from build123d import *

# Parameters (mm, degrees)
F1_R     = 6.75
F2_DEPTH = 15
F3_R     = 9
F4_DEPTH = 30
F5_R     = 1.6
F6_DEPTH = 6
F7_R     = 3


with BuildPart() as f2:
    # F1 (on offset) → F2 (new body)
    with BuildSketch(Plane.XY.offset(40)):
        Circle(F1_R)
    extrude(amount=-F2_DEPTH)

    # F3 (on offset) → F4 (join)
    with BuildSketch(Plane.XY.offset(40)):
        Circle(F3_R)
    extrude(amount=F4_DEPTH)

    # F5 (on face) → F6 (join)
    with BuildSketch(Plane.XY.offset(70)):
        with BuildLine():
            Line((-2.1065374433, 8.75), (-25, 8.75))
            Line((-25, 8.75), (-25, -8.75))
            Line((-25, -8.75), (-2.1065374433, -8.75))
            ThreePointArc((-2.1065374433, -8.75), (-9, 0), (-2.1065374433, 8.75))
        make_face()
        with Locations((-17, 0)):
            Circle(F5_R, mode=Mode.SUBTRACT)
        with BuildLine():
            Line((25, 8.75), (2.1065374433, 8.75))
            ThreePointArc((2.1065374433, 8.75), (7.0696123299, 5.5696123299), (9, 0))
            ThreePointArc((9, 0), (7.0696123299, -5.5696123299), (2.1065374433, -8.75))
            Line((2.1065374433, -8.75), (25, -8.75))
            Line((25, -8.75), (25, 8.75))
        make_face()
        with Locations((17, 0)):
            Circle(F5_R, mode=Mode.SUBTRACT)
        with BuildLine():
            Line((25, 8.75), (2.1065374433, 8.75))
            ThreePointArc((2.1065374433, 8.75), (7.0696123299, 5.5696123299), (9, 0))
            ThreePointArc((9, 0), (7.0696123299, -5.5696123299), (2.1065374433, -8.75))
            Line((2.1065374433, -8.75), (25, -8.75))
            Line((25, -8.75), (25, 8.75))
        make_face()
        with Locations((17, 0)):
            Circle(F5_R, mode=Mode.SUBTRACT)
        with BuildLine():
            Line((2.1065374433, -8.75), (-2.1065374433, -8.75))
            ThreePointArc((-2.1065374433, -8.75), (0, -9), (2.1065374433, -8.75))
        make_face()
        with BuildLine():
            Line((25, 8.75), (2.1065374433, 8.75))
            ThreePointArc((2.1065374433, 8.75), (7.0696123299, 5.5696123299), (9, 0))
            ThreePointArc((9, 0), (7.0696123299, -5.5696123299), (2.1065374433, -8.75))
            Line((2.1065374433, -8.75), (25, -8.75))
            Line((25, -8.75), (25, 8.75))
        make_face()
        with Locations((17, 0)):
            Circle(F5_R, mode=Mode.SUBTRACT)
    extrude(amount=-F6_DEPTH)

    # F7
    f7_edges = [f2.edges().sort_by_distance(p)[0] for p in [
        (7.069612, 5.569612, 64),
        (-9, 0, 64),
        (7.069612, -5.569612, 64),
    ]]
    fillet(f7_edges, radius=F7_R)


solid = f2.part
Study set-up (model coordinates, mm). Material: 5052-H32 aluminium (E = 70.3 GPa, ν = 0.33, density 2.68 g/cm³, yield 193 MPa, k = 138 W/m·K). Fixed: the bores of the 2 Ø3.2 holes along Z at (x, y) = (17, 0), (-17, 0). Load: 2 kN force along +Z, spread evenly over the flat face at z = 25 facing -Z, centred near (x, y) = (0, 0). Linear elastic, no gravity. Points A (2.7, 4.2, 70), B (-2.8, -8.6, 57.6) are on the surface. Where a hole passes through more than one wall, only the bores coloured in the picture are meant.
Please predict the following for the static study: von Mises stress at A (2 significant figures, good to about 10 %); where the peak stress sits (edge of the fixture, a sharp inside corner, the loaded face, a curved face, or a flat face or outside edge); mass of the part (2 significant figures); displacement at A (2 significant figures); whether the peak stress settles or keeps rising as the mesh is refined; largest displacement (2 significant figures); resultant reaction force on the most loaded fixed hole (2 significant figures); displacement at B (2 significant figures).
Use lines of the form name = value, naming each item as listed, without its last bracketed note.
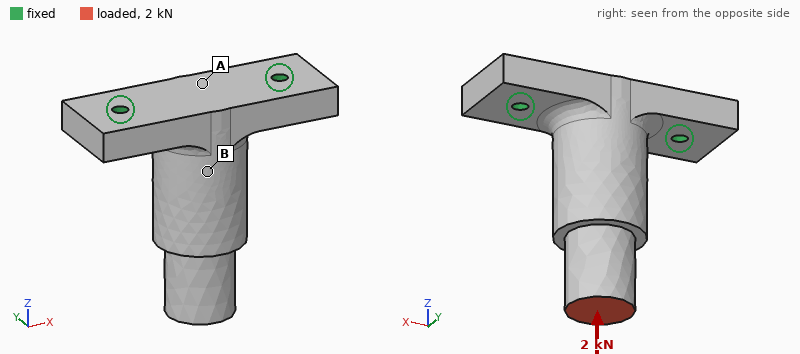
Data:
von Mises stress at A = 18 MPa
where the peak stress sits = edge of the fixture
mass of the part = 36 g
displacement at A = 11 µm
whether the peak stress settles or keeps rising as the mesh is refined = keeps rising
largest displacement = 16 µm
resultant reaction force on the most loaded fixed hole = 1.1 kN
displacement at B = 11 µm
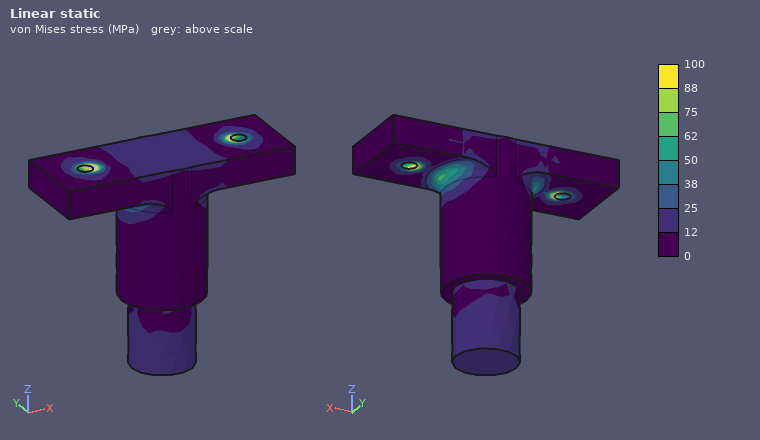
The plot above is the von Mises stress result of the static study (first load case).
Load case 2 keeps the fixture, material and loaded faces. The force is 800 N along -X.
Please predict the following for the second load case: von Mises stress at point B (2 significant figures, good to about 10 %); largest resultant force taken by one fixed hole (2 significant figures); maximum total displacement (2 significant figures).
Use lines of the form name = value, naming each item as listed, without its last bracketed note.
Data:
von Mises stress at point B = 13 MPa
largest resultant force taken by one fixed hole = 1.3 kN
maximum total displacement = 96 µm
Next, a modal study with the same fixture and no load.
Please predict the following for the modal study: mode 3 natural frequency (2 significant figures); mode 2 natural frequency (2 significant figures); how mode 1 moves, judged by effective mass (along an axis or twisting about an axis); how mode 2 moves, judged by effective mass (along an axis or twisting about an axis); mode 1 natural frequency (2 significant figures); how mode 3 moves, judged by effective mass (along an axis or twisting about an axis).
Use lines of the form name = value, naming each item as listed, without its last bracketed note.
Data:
mode 3 natural frequency = 12 kHz
mode 2 natural frequency = 6600 Hz
how mode 1 moves, judged by effective mass = along Y
how mode 2 moves, judged by effective mass = along X
mode 1 natural frequency = 3200 Hz
how mode 3 moves, judged by effective mass = along Z
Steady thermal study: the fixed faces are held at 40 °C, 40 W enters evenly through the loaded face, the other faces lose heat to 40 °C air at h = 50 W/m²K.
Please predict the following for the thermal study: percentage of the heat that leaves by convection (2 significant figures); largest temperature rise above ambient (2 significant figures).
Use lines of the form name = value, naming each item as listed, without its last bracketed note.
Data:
percentage of the heat that leaves by convection = 12 %
largest temperature rise above ambient = 72 K
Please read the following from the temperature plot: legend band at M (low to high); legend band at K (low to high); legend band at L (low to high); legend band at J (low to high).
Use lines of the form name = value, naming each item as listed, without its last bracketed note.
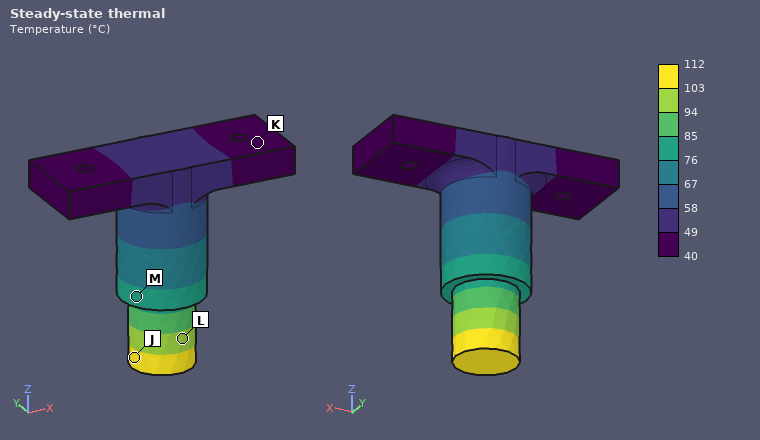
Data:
legend band at M = 76 to 85 °C
legend band at K = 40 to 49 °C
legend band at L = 94 to 103 °C
legend band at J = 103 to 112 °C
